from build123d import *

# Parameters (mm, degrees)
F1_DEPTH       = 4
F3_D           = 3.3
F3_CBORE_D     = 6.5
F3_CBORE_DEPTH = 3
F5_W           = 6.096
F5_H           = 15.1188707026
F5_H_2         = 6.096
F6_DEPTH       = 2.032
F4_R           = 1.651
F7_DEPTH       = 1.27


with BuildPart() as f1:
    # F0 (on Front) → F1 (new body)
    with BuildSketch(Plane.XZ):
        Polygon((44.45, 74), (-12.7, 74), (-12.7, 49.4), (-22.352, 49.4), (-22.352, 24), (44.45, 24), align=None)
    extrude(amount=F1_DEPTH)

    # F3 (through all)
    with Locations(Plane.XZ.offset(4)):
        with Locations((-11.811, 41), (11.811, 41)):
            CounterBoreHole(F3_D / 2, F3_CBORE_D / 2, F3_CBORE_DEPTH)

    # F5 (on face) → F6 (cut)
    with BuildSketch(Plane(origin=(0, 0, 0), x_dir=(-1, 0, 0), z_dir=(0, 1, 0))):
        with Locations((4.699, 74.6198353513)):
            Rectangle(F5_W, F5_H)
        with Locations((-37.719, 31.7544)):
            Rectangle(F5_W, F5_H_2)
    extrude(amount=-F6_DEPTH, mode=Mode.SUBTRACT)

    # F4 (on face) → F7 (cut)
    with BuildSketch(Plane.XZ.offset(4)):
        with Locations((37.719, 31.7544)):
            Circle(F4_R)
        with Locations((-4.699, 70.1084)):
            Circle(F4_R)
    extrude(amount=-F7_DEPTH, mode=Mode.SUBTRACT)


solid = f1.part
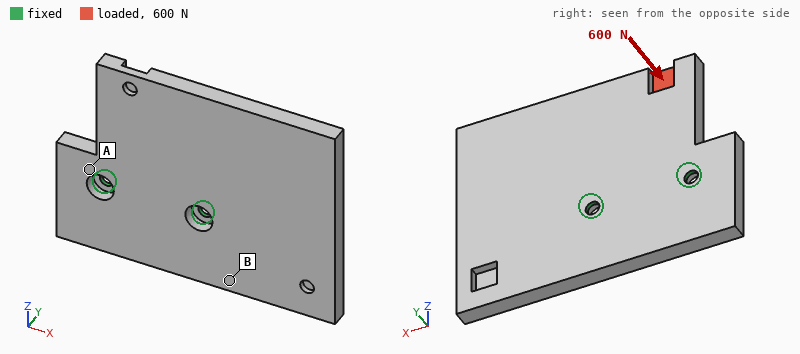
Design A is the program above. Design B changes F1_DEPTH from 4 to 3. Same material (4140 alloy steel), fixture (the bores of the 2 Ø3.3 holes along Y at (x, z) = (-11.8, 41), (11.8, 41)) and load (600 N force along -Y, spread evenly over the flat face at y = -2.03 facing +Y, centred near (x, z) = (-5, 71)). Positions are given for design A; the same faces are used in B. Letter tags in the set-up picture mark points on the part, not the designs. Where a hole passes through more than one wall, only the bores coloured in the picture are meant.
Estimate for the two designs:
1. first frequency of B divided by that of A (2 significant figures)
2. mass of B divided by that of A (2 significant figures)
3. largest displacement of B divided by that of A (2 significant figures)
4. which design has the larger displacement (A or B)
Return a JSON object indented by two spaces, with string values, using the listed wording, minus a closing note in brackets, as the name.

{
  "first frequency of B divided by that of A": "0.97",
  "mass of B divided by that of A": "0.75",
  "largest displacement of B divided by that of A": "1.5",
  "which design has the larger displacement": "B"
}
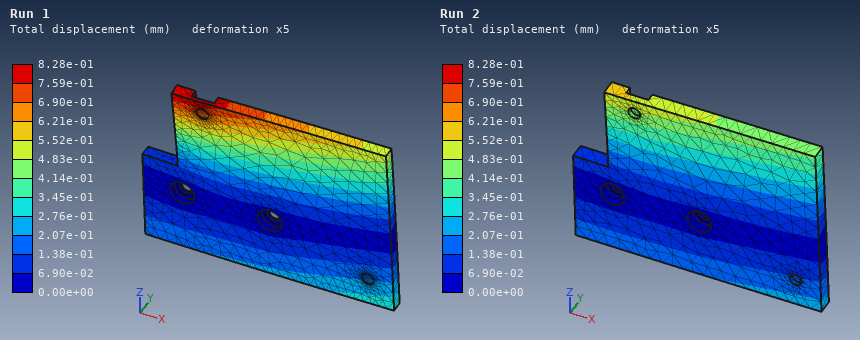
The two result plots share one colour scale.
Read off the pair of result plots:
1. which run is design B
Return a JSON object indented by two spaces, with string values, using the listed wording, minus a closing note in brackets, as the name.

{
  "which run is design B": "Run 1"
}
